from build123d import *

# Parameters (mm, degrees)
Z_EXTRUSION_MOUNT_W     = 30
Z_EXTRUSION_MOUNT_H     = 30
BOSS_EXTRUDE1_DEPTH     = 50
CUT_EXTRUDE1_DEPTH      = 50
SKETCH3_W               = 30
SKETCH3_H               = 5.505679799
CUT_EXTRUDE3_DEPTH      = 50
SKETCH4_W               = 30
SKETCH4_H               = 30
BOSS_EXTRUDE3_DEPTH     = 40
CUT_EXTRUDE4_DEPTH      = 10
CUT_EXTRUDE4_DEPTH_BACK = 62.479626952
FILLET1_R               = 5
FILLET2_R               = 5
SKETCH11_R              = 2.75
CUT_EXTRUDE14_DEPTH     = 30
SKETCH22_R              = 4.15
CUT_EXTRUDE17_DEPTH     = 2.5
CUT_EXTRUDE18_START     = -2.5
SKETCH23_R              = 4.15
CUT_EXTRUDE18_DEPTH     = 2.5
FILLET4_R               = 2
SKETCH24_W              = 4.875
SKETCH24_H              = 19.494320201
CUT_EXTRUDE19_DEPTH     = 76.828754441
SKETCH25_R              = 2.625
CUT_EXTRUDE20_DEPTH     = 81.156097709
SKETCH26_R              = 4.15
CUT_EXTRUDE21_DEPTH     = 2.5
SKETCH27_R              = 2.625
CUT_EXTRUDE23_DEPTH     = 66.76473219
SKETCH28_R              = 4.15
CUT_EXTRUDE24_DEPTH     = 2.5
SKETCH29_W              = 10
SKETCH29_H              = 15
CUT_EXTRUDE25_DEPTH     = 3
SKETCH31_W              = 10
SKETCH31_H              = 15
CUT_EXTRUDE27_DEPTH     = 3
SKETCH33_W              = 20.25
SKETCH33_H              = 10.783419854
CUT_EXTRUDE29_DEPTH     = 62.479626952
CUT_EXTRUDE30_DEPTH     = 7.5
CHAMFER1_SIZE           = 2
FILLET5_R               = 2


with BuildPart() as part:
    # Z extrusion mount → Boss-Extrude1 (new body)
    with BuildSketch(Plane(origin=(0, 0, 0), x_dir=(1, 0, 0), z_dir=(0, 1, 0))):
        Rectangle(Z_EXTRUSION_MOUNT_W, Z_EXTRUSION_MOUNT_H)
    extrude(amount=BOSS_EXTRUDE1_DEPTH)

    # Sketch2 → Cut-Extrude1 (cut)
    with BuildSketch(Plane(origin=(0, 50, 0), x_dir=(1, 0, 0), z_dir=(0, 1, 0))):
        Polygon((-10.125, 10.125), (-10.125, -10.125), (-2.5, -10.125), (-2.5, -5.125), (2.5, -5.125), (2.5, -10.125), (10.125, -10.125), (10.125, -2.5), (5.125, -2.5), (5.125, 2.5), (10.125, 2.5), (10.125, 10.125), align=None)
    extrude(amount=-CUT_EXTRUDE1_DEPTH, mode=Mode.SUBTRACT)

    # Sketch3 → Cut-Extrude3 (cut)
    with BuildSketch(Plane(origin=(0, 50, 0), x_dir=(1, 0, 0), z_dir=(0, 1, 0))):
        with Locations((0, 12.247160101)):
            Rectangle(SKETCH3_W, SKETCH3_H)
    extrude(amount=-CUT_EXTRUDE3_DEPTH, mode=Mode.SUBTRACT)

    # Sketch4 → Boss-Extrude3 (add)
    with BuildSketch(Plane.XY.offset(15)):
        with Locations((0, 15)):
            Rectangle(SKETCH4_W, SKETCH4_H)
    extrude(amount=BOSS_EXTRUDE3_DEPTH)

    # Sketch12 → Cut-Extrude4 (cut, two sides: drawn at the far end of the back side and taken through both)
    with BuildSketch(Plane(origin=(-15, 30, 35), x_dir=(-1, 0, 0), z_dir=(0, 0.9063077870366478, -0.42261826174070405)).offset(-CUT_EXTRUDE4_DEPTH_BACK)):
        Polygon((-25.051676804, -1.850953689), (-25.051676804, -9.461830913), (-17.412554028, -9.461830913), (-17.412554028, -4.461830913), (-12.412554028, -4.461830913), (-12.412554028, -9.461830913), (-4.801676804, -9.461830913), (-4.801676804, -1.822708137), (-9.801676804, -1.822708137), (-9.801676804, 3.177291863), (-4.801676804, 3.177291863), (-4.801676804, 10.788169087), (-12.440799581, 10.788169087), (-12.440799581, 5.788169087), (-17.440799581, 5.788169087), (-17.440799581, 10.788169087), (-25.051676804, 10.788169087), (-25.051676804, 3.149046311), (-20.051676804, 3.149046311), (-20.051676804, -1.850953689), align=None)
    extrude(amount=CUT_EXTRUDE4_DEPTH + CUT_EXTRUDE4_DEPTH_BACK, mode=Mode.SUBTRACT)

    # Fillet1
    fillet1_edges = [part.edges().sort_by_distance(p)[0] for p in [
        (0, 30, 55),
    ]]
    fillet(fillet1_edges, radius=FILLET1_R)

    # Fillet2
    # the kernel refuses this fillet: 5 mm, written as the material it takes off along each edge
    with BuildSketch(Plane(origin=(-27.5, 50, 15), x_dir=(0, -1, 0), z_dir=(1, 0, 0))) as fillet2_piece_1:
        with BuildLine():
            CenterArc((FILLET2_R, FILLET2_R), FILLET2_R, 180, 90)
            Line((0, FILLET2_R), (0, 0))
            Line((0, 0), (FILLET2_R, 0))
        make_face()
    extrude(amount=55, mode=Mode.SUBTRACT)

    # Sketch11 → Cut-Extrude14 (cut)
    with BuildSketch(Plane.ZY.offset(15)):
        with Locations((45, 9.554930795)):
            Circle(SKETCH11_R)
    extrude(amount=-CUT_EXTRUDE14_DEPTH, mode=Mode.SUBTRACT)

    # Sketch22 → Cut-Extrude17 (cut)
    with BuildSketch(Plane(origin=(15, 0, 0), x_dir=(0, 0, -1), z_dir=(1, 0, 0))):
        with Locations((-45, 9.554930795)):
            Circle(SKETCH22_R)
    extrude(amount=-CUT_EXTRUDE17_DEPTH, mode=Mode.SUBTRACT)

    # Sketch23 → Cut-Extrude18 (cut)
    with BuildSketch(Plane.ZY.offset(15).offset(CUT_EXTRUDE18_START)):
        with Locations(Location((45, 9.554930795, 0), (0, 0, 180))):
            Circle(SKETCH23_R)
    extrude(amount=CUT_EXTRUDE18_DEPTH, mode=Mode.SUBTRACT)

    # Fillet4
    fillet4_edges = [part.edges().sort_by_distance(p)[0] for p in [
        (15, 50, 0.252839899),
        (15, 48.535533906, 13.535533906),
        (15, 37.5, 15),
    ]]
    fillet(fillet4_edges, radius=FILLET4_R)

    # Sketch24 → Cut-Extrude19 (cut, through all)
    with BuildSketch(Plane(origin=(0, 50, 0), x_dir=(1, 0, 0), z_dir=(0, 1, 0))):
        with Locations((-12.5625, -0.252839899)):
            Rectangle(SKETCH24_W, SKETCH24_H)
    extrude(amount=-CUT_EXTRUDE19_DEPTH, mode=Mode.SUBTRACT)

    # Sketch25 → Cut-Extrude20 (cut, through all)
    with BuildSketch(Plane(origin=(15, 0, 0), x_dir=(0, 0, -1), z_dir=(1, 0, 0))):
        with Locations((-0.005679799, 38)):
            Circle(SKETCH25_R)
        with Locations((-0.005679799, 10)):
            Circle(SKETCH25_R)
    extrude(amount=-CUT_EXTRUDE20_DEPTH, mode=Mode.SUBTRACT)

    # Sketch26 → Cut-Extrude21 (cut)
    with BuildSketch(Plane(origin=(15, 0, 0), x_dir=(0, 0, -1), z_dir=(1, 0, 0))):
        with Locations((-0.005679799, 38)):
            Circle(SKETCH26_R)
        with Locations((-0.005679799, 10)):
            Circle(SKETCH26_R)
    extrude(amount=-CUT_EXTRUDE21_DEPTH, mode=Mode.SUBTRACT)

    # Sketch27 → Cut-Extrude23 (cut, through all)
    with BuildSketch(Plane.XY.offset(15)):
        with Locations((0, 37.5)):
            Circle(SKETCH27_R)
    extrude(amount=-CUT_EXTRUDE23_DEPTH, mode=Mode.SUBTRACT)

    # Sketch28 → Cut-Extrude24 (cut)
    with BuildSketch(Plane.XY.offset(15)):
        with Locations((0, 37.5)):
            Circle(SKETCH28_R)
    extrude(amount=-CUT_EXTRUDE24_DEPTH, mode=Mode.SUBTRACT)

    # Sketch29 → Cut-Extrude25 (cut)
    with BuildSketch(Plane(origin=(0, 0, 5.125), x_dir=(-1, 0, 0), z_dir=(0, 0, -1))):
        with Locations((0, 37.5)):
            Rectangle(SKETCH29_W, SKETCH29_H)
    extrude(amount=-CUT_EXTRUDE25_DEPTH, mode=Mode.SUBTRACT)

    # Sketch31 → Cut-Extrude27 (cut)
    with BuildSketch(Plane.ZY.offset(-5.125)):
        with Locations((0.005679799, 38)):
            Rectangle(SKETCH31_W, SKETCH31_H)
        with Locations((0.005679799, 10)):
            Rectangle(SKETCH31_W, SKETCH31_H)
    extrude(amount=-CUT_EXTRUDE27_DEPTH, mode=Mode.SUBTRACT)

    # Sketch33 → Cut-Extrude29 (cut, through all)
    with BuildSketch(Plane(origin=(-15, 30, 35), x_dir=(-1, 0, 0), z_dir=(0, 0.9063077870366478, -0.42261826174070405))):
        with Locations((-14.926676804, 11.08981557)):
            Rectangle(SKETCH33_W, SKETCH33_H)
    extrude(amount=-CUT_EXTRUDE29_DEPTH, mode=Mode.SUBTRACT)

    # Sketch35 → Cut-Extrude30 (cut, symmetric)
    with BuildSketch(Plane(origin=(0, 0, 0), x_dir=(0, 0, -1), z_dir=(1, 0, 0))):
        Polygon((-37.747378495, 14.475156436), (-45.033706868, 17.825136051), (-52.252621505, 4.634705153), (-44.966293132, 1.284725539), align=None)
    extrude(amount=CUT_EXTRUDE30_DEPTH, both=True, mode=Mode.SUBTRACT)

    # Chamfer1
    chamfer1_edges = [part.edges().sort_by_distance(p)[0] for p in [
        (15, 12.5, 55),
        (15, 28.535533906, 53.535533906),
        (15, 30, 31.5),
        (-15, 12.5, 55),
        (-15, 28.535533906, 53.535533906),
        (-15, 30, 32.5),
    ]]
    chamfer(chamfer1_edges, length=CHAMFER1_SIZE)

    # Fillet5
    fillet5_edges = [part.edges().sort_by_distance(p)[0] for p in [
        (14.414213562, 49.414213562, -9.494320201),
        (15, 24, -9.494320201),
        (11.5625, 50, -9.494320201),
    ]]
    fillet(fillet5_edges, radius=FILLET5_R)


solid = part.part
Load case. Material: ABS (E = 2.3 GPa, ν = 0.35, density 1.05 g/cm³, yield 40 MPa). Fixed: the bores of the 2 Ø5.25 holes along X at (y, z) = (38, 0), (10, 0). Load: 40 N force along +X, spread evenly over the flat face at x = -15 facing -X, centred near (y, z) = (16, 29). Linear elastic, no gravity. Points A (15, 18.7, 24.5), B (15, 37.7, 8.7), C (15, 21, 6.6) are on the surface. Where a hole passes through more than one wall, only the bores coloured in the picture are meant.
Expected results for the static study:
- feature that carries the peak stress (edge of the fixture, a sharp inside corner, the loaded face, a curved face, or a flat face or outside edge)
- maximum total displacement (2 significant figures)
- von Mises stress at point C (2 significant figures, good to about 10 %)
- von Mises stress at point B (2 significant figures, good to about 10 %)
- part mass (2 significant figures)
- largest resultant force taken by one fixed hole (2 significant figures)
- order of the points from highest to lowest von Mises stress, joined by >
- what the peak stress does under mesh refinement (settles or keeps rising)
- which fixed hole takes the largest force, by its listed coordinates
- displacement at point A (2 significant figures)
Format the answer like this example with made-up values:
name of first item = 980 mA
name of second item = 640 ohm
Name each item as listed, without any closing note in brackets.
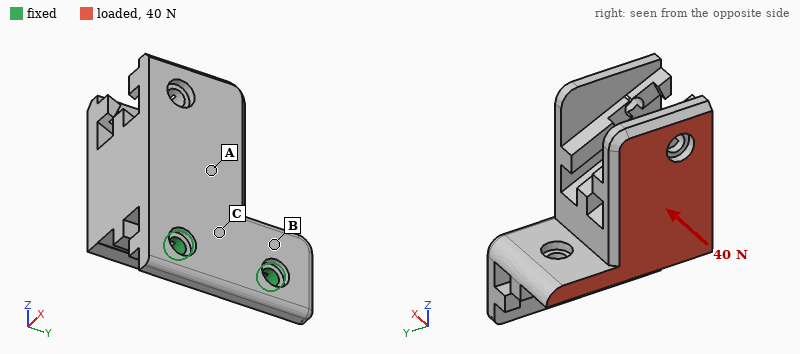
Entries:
feature that carries the peak stress = edge of the fixture
maximum total displacement = 0.98 mm
von Mises stress at point C = 4.6 MPa
von Mises stress at point B = 2.6 MPa
part mass = 38 g
largest resultant force taken by one fixed hole = 30 N
order of the points from highest to lowest von Mises stress, joined by > = C > B > A
what the peak stress does under mesh refinement = keeps rising
which fixed hole takes the largest force, by its listed coordinates = (10, 0)
displacement at point A = 0.34 mm
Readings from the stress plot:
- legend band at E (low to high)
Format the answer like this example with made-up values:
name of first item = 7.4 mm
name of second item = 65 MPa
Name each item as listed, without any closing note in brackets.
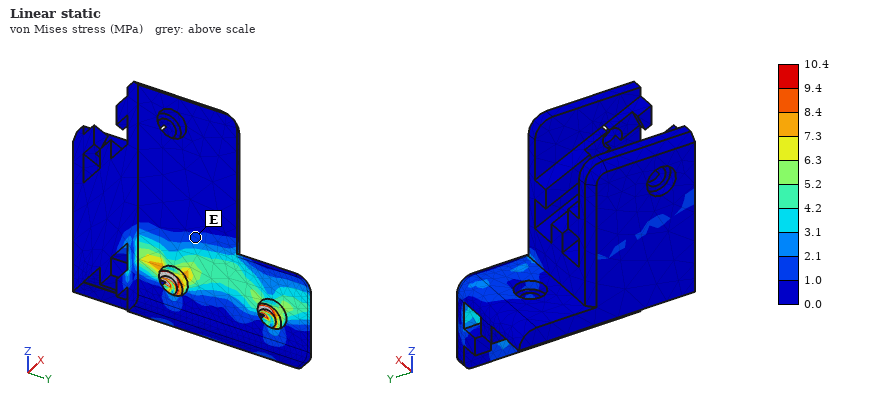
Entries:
legend band at E = 1.0 to 2.1 MPa
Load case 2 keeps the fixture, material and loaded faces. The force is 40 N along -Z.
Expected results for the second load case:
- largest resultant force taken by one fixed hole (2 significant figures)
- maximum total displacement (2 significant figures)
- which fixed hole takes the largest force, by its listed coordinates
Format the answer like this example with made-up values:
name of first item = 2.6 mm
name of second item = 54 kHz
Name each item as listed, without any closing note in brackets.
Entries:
largest resultant force taken by one fixed hole = 31 N
maximum total displacement = 1.0 mm
which fixed hole takes the largest force, by its listed coordinates = (10, 0)
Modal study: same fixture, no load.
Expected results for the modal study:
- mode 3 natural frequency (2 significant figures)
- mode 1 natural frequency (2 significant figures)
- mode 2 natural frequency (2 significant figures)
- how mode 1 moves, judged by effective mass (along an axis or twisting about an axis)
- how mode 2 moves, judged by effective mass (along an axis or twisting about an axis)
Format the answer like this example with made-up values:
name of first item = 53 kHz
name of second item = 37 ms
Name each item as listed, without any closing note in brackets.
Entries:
mode 3 natural frequency = 1700 Hz
mode 1 natural frequency = 240 Hz
mode 2 natural frequency = 970 Hz
how mode 1 moves, judged by effective mass = along X
how mode 2 moves, judged by effective mass = along Y
